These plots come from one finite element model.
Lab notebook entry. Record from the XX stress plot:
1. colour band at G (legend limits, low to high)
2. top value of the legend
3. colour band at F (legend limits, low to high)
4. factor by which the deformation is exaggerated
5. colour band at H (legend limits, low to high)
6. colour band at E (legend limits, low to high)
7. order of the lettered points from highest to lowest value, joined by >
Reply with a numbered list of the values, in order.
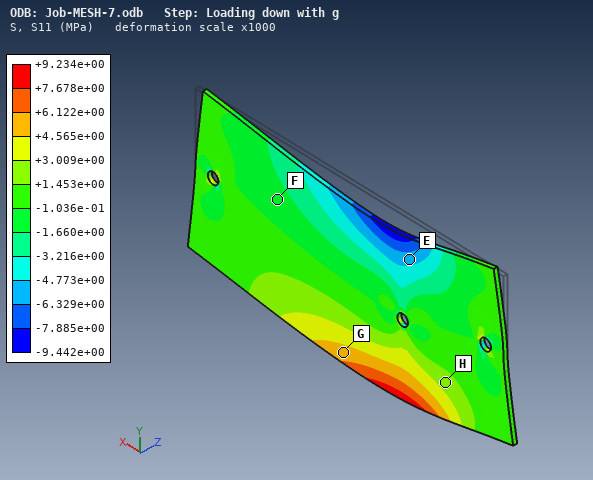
1. +4.565e+00 to +6.122e+00 MPa
2. +9.234e+00 MPa
3. -1.660e+00 to -1.036e-01 MPa
4. 1000
5. +1.453e+00 to +3.009e+00 MPa
6. -6.329e+00 to -4.773e+00 MPa
7. G > H > F > E
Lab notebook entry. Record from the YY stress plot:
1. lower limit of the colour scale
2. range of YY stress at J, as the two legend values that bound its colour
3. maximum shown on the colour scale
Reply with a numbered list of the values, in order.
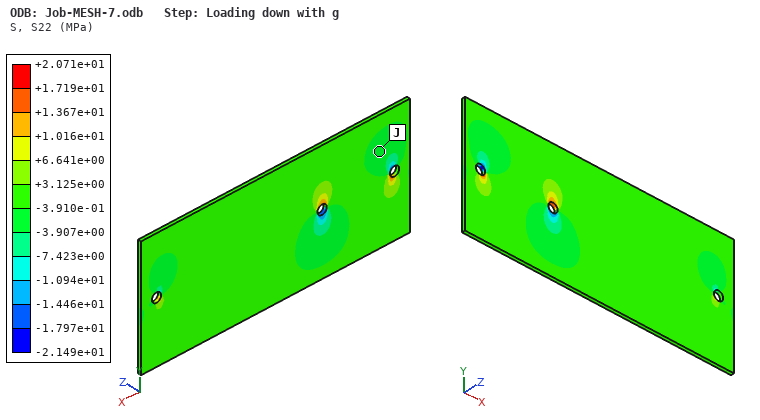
1. -2.149e+01 MPa
2. -3.907e+00 to -3.910e-01 MPa
3. +2.071e+01 MPa
